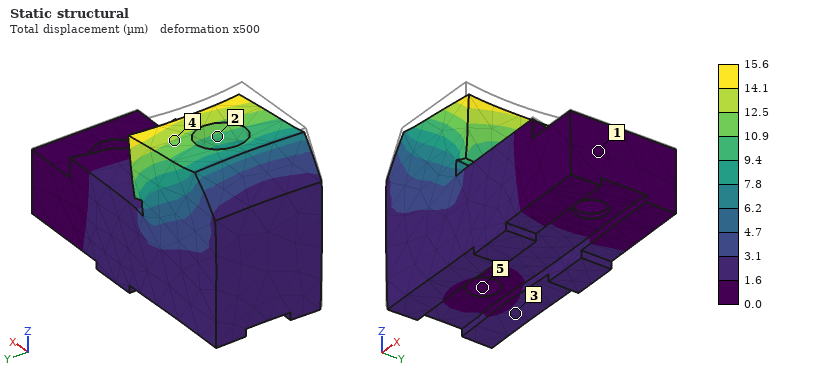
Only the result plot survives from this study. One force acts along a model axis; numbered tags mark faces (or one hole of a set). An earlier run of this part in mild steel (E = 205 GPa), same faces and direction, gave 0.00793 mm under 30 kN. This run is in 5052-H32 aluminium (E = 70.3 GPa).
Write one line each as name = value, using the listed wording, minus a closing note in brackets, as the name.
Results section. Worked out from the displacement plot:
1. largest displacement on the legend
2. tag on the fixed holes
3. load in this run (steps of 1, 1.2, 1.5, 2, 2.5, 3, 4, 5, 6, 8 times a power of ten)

largest displacement on the legend = 15.6 µm
tag on the fixed holes = 5
load in this run = 20 kN
